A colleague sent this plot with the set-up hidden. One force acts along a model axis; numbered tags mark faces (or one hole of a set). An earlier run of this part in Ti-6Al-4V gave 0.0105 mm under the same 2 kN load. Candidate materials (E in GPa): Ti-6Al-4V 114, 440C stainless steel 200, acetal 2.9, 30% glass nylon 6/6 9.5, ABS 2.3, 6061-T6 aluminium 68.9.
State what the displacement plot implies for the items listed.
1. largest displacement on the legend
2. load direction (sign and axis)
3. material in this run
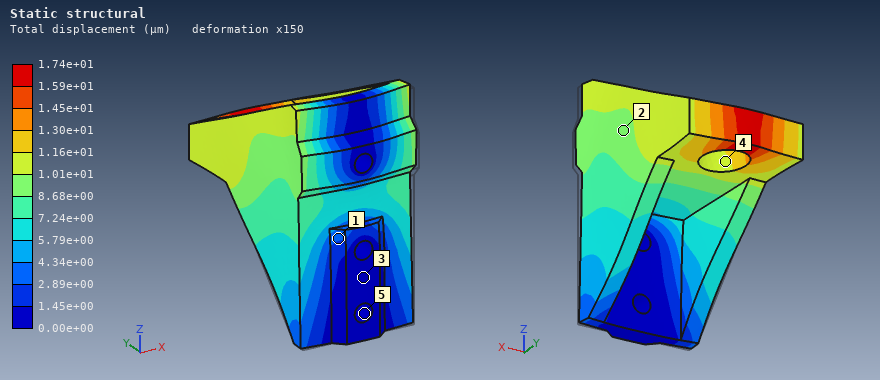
1.74e+01 µm
+Y
6061-T6 aluminium
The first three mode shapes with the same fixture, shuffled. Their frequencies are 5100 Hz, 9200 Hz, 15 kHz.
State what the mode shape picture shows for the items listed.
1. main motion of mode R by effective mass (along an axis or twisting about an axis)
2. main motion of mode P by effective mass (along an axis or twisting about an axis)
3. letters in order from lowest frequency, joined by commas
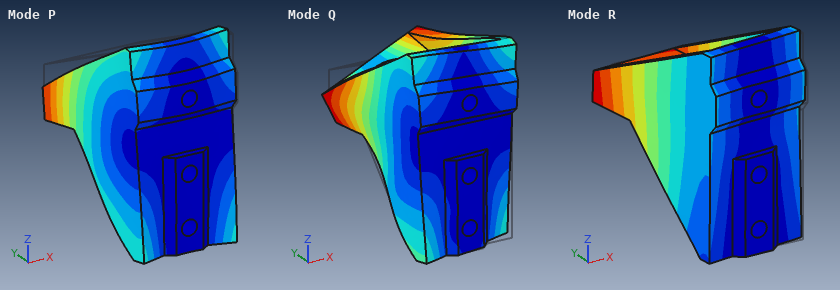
along X
along Z
R, P, Q
